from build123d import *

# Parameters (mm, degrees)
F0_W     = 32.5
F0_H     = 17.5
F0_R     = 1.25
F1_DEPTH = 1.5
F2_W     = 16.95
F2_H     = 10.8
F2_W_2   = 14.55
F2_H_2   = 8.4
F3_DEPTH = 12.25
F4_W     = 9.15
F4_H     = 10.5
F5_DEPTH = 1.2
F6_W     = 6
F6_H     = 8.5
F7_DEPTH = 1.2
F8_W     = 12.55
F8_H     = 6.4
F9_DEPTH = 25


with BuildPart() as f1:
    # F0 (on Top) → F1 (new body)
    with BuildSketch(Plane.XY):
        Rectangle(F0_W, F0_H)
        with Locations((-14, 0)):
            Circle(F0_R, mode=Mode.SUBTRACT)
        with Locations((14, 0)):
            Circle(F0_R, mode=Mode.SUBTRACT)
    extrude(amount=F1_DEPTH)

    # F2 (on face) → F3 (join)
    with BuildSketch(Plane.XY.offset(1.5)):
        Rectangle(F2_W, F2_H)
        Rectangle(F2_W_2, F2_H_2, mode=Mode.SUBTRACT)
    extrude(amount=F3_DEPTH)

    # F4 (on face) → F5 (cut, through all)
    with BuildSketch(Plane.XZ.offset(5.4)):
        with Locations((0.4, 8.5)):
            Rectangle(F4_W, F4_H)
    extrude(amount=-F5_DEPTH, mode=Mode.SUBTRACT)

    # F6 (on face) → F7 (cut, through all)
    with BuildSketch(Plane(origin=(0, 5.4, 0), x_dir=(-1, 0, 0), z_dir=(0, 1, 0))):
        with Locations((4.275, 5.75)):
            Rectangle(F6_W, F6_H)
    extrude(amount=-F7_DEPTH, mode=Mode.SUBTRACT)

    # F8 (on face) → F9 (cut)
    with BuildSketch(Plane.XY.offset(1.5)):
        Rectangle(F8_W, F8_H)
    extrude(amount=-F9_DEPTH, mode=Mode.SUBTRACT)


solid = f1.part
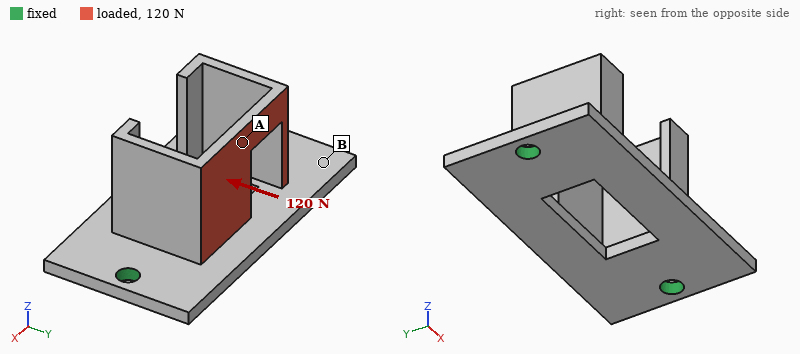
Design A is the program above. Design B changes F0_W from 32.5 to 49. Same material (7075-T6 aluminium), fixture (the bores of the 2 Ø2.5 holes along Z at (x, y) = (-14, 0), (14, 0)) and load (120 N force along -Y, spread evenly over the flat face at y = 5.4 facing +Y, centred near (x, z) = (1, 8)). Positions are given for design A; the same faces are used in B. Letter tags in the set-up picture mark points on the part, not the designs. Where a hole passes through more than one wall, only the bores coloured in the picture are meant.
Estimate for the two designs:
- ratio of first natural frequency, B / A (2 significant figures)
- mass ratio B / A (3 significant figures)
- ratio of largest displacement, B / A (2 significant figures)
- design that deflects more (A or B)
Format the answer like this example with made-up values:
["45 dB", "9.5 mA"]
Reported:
["1.1", "1.34", "0.87", "A"]
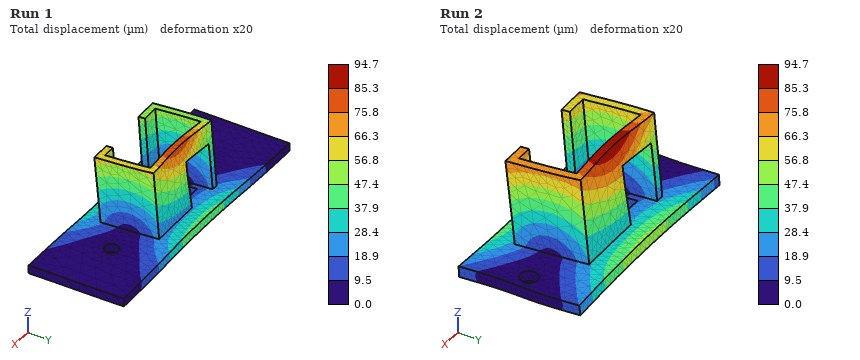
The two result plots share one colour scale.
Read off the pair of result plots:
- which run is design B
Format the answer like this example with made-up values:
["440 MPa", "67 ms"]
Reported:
["Run 1"]
